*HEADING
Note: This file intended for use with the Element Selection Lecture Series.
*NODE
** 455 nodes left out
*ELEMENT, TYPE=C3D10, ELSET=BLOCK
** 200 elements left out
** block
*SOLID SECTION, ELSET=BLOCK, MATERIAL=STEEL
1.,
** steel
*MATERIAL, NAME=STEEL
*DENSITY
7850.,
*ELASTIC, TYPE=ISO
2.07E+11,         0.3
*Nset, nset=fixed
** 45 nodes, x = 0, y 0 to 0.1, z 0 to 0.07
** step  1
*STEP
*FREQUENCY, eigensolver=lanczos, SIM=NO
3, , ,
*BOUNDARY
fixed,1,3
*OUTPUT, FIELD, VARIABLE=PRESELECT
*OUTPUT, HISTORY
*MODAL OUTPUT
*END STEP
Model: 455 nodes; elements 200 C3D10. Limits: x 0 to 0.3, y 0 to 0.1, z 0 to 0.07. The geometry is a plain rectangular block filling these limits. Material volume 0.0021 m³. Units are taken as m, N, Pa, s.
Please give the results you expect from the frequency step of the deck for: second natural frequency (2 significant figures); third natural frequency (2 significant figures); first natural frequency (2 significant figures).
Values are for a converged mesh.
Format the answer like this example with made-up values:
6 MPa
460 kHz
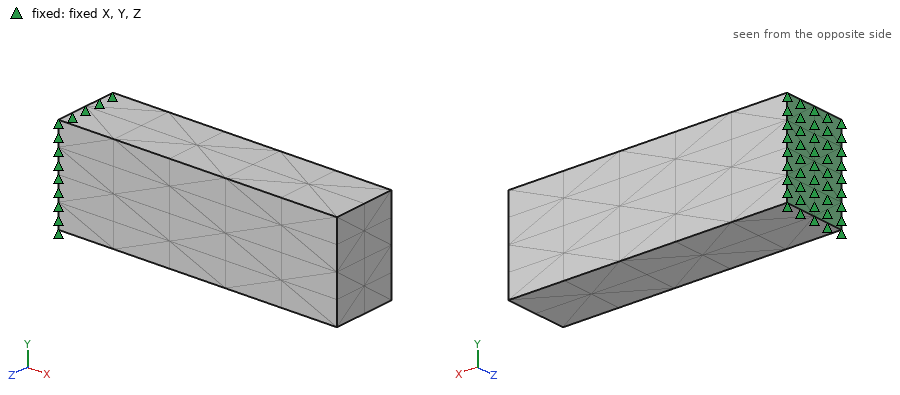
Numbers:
860 Hz
2300 Hz
630 Hz
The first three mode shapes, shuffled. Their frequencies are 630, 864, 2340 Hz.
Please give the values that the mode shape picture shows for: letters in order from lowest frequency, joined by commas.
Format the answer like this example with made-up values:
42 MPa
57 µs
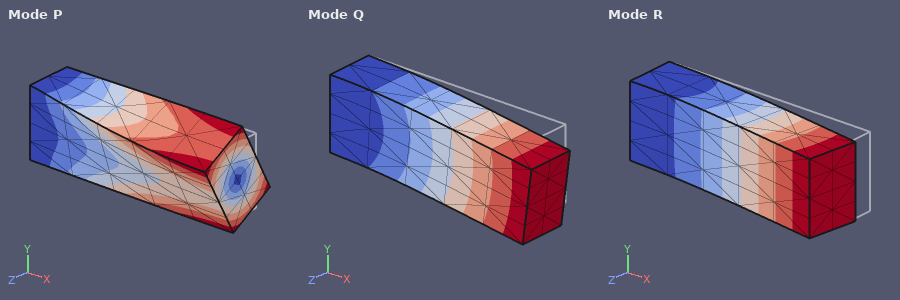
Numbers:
R, Q, P
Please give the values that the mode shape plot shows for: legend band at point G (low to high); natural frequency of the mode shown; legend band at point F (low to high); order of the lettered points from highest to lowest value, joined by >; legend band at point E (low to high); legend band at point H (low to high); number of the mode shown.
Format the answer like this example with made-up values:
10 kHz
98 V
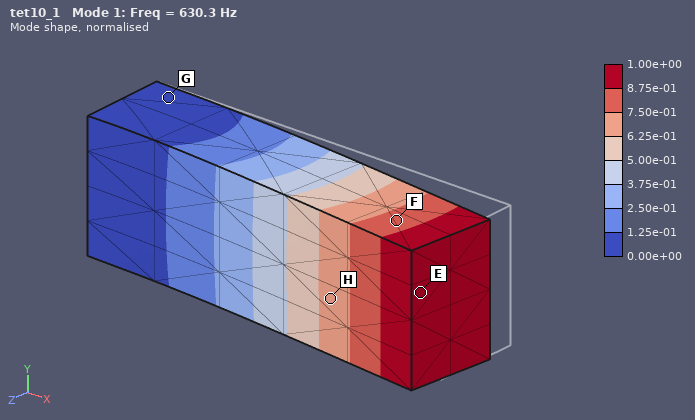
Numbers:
0.00e+00 to 1.25e-01
630.3 Hz
7.50e-01 to 8.75e-01
E > F > H > G
8.75e-01 to 1.00e+00
6.25e-01 to 7.50e-01
1
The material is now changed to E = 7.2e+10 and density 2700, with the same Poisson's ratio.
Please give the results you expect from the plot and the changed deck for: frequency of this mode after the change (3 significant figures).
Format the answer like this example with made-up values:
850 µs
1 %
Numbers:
634 Hz
